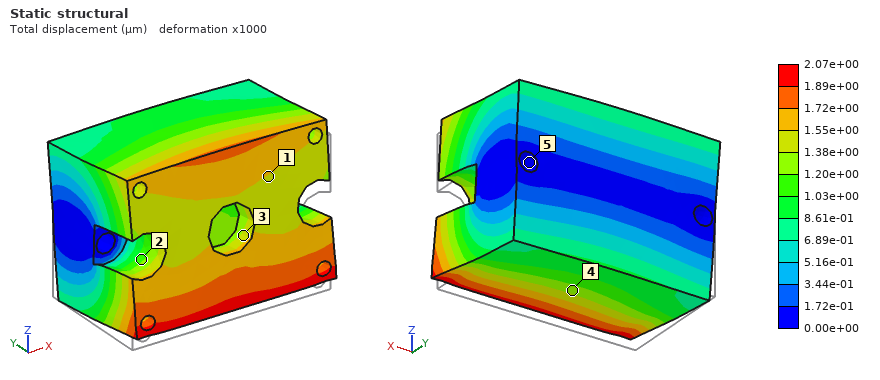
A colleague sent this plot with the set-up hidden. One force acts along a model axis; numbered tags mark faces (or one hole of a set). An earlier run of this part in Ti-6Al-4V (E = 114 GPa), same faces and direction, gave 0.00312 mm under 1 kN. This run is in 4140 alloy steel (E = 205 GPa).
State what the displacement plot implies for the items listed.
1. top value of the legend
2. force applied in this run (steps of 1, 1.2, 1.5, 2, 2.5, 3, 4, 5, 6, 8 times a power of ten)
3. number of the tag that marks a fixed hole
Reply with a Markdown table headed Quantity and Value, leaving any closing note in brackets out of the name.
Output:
| Quantity | Value |
|---|---|
| top value of the legend | 2.07e+00 µm |
| force applied in this run | 1.2 kN |
| number of the tag that marks a fixed hole | 5 |
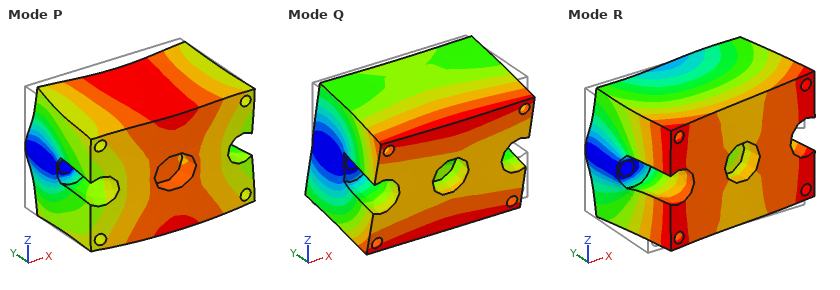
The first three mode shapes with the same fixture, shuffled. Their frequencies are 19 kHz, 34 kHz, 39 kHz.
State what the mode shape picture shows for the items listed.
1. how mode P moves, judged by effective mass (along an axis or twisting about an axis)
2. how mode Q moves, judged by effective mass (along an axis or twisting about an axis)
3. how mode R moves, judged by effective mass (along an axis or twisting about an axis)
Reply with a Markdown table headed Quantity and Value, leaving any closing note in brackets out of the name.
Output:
| Quantity | Value |
|---|---|
| how mode P moves, judged by effective mass | along Y |
| how mode Q moves, judged by effective mass | along Z |
| how mode R moves, judged by effective mass | along X |
